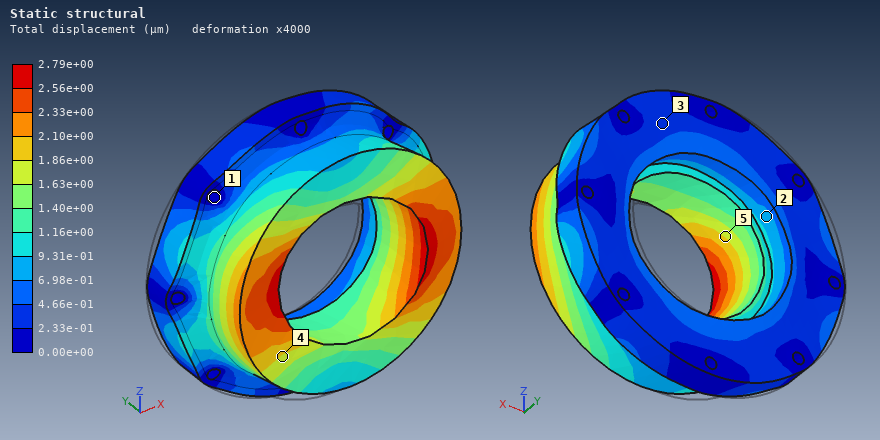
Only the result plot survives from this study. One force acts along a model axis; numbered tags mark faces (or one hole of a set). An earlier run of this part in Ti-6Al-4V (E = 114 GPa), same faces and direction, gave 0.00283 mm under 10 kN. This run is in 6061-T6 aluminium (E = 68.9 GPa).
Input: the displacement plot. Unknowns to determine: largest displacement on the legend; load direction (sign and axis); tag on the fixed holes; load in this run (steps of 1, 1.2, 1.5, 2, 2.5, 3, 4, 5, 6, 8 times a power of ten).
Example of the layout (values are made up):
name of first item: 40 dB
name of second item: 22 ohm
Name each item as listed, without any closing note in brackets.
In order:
largest displacement on the legend: 2.79e+00 µm
load direction: +X
tag on the fixed holes: 1
load in this run: 6 kN
